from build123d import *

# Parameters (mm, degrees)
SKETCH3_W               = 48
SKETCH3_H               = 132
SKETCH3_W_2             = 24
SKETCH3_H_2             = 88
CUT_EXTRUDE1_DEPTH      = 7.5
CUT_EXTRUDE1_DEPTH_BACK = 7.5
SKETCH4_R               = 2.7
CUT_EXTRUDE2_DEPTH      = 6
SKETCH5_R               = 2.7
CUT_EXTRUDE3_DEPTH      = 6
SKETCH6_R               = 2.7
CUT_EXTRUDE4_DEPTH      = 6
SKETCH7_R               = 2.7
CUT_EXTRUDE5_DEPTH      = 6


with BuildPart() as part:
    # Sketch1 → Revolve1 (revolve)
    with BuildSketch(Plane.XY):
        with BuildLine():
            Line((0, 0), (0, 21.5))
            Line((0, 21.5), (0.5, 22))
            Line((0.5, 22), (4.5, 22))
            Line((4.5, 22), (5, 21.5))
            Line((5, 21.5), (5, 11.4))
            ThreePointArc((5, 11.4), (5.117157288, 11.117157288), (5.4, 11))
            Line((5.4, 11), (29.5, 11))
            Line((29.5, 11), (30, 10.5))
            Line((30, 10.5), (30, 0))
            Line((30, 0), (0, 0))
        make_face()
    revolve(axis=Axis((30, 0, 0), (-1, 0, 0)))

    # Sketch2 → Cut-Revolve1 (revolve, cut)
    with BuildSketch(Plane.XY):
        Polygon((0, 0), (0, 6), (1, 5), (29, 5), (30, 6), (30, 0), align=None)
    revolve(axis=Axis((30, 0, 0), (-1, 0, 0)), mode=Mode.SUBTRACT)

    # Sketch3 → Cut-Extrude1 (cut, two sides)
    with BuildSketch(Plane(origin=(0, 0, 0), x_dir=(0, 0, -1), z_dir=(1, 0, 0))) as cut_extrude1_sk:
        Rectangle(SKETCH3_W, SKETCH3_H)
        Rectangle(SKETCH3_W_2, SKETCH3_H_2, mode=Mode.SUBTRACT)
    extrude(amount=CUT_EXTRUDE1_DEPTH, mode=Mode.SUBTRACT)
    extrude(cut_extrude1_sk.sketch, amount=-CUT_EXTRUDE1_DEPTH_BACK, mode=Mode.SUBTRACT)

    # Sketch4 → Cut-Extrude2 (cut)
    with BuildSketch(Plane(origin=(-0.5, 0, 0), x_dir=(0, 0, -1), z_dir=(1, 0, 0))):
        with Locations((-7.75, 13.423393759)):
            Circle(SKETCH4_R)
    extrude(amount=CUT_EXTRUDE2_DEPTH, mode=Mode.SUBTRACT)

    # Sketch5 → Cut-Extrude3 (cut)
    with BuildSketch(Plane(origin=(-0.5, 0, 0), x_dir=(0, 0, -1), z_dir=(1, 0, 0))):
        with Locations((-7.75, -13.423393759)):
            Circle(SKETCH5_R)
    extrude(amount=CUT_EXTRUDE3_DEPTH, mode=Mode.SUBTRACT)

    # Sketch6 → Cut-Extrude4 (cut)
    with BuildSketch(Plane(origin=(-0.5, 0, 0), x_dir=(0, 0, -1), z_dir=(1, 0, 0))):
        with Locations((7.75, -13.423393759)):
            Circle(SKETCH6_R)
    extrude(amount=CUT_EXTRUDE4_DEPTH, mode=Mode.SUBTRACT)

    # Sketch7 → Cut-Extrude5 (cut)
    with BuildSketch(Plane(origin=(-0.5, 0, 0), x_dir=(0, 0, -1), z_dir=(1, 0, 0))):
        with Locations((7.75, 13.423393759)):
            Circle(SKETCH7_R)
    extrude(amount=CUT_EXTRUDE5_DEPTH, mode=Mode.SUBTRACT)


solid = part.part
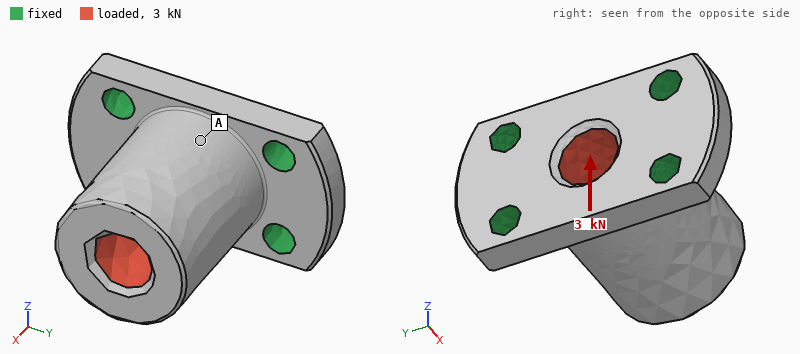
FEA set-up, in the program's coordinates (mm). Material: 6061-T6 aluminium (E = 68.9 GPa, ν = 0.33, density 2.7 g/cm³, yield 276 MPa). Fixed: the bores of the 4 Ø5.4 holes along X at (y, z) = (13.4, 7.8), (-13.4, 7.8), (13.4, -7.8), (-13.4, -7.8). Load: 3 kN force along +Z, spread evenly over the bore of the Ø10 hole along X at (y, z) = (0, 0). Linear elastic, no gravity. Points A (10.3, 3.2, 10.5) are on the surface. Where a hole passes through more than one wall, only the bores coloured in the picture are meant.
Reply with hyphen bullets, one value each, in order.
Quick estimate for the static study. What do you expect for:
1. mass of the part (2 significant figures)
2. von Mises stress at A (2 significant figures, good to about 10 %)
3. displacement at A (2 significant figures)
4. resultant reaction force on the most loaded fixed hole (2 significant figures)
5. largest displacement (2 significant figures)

- 31 g
- 15 MPa
- 18 µm
- 1.5 kN
- 45 µm
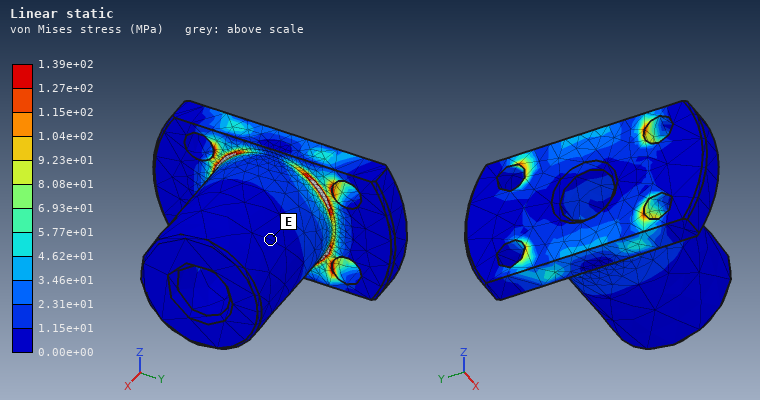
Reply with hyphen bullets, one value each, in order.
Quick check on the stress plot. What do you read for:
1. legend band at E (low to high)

- 0.00e+00 to 1.15e+01 MPa
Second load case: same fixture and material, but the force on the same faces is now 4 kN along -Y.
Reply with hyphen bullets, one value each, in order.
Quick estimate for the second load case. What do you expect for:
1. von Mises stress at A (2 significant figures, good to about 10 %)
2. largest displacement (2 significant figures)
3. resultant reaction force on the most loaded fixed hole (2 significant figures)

- 17 MPa
- 31 µm
- 1.6 kN
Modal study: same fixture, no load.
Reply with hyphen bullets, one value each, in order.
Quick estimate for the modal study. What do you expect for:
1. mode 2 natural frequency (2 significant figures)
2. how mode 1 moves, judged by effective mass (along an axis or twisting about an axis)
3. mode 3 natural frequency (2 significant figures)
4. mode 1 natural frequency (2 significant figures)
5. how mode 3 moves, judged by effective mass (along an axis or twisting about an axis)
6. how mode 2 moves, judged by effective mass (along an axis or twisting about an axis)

- 14 kHz
- along Z
- 25 kHz
- 9800 Hz
- along X
- along Y
